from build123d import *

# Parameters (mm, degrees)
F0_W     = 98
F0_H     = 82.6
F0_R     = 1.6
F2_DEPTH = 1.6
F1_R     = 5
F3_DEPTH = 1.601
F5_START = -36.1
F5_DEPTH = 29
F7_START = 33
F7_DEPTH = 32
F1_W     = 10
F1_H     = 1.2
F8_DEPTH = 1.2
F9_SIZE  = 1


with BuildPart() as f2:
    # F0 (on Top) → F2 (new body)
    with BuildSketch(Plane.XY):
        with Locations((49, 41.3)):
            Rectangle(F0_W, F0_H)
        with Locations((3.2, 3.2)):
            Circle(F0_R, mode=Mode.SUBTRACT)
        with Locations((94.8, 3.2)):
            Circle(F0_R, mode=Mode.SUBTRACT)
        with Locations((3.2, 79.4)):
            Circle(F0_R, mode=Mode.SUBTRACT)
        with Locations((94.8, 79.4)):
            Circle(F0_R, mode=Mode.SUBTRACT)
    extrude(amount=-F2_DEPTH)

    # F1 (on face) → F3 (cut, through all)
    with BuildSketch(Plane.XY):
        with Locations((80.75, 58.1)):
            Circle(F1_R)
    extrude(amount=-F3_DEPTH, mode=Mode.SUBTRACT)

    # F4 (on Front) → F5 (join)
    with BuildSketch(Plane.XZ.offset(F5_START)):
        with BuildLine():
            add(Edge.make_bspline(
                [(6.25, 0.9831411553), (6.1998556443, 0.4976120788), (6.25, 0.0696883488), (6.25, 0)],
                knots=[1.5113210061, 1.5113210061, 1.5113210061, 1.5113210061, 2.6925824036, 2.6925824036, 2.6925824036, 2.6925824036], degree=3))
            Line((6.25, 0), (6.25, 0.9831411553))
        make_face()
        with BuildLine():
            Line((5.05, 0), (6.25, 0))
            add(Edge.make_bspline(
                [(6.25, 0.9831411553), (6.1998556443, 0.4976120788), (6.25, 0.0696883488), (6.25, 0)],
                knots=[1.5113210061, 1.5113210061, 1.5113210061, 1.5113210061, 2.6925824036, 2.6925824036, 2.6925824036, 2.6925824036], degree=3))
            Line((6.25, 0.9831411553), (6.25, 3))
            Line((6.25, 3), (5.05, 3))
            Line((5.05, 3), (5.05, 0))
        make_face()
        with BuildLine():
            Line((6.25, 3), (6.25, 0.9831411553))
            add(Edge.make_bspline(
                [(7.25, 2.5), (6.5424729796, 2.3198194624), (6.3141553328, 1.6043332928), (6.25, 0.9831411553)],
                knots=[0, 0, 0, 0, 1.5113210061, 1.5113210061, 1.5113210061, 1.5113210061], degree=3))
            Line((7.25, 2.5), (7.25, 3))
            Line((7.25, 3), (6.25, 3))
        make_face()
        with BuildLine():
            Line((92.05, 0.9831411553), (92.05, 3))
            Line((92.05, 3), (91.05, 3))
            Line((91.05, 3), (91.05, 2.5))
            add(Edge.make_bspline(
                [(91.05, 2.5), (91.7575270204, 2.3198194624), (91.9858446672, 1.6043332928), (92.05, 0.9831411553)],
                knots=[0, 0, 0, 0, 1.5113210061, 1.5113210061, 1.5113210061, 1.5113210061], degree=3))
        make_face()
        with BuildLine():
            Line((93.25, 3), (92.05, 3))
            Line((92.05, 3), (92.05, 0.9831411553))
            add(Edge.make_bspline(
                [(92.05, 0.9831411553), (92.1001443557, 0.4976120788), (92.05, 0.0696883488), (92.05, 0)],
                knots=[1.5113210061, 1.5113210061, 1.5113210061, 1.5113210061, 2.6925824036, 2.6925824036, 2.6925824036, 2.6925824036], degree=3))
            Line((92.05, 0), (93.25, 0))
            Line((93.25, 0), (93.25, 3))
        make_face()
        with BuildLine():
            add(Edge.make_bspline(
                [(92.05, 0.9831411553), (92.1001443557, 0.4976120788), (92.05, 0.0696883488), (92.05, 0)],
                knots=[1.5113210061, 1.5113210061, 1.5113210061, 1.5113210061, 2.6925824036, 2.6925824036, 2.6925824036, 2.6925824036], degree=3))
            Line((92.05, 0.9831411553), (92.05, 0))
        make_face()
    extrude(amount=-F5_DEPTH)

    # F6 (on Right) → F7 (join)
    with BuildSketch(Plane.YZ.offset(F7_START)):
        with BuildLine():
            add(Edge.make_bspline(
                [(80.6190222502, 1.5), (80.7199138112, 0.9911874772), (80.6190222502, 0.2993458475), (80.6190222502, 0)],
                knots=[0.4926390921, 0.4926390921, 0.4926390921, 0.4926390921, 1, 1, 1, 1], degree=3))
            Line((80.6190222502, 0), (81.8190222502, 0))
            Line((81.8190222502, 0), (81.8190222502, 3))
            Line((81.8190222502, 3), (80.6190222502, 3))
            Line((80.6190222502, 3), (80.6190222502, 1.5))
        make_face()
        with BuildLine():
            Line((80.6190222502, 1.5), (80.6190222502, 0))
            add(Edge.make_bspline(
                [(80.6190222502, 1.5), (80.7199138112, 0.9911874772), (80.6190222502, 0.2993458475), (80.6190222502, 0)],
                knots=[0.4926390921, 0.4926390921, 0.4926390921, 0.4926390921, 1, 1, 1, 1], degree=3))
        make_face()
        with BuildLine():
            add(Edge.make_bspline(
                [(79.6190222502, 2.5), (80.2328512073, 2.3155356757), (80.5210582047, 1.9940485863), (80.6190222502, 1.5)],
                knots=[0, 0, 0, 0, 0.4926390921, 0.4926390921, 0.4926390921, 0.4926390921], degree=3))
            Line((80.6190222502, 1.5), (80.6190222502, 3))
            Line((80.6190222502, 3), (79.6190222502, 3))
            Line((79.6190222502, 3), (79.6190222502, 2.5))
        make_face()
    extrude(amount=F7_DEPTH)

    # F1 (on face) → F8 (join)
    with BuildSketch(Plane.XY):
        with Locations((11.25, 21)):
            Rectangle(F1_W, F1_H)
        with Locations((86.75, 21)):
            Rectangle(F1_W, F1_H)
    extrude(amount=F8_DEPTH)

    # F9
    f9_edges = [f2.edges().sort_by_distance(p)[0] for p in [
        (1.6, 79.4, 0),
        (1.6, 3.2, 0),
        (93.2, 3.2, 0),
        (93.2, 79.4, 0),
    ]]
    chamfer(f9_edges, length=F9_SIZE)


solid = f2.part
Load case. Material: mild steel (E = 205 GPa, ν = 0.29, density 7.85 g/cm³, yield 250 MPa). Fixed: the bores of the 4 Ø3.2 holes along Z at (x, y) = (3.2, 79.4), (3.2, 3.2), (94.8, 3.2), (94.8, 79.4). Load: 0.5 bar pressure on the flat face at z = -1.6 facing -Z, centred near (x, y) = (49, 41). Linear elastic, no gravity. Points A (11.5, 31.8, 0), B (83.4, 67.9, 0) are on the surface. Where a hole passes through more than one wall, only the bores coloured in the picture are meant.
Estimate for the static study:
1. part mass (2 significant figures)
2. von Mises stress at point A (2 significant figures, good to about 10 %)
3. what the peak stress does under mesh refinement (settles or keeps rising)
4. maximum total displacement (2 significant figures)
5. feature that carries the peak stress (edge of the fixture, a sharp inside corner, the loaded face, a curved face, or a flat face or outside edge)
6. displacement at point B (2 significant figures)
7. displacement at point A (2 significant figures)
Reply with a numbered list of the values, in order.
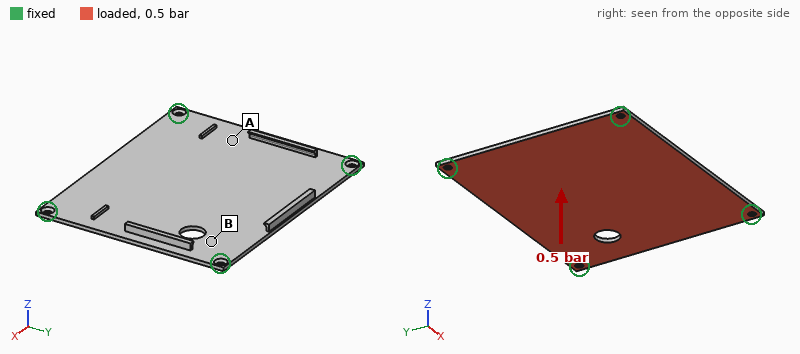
1. 100 g
2. 54 MPa
3. keeps rising
4. 0.32 mm
5. edge of the fixture
6. 0.11 mm
7. 0.15 mm
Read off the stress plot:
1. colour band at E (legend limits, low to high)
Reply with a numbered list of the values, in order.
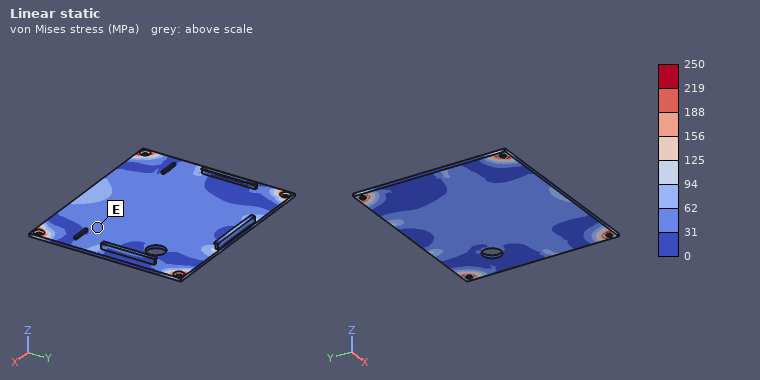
1. 31 to 62 MPa
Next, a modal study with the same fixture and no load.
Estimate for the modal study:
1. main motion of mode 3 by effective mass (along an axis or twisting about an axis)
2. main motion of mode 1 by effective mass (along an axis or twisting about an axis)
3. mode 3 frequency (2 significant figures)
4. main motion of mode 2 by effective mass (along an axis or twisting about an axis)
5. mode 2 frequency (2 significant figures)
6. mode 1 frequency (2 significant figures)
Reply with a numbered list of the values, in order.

1. twisting about Y
2. along Z
3. 1400 Hz
4. twisting about X
5. 1200 Hz
6. 670 Hz
